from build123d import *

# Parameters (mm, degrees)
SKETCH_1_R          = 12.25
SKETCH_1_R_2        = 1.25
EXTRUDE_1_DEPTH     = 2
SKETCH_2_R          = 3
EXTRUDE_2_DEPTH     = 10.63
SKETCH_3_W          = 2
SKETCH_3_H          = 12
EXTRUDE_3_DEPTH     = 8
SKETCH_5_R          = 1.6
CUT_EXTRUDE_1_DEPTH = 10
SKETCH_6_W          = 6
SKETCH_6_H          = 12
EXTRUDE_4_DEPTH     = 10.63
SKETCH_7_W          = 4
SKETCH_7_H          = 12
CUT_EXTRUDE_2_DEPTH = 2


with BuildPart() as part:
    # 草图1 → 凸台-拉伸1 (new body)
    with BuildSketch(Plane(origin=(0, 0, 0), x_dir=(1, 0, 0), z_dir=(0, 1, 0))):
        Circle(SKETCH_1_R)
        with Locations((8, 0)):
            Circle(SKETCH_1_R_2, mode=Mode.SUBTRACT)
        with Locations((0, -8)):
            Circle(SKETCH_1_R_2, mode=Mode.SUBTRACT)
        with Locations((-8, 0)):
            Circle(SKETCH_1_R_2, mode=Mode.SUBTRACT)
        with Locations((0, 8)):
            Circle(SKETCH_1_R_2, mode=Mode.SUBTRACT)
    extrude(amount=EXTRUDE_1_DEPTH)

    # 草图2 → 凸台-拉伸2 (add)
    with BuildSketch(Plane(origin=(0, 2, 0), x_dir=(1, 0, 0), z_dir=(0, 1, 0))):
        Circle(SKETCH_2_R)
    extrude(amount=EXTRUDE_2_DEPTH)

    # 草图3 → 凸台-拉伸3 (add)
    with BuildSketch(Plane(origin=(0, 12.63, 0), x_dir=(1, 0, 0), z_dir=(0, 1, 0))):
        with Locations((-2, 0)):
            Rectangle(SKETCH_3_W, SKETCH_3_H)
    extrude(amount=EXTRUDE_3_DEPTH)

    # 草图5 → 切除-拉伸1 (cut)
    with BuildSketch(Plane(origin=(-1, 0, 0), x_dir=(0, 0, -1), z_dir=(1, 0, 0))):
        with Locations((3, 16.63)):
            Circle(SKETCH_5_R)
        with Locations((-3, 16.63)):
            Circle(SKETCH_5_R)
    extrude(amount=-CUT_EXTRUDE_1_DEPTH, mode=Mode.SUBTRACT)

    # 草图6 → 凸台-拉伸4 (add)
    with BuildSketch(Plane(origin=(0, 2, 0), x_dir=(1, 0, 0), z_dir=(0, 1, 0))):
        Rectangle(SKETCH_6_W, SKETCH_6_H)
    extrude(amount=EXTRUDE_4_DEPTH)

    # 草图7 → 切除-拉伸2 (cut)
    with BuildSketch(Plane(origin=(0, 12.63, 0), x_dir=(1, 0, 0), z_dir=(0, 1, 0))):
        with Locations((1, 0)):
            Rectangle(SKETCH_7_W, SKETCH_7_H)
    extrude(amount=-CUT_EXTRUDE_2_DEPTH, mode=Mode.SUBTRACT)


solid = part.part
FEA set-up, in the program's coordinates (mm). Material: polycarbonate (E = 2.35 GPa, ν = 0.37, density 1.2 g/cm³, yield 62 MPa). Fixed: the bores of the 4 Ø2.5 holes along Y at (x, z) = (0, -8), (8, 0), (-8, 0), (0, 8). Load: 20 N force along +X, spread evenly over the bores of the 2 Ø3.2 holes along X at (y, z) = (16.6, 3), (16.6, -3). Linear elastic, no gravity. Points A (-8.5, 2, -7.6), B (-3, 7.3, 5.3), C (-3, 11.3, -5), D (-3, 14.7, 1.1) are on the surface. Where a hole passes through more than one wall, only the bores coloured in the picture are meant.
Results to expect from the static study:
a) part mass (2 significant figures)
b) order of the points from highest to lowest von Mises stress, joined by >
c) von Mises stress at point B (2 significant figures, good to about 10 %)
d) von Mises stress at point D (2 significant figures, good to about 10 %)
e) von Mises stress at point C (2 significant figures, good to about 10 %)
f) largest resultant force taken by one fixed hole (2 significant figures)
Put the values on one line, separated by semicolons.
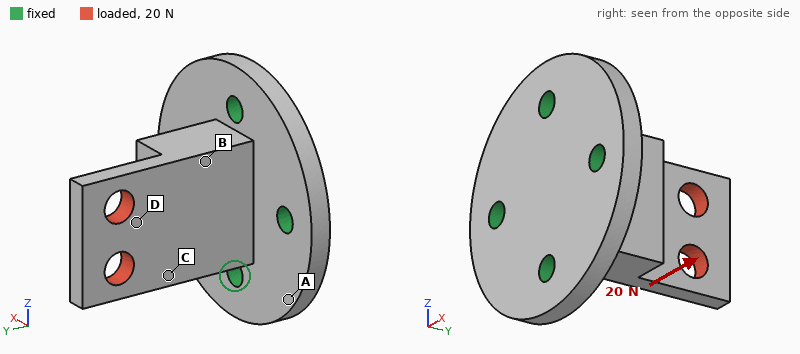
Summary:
2.1 g; C > D > B > A; 3.3 MPa; 6.1 MPa; 11 MPa; 20 N
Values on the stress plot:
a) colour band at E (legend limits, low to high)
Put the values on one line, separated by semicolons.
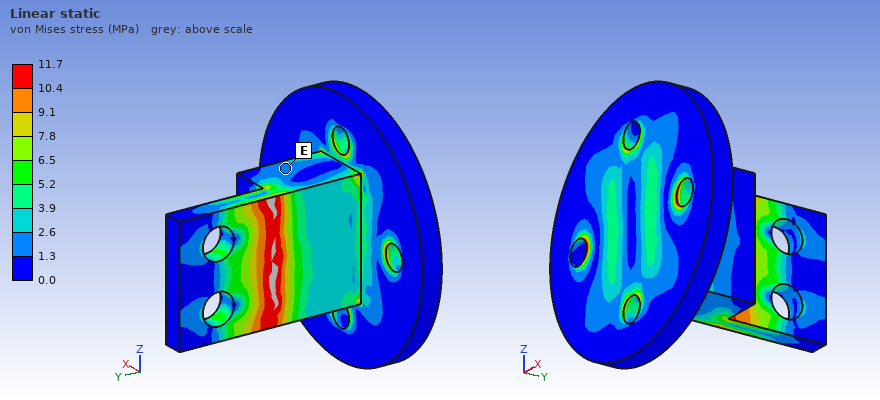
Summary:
1.3 to 2.6 MPa
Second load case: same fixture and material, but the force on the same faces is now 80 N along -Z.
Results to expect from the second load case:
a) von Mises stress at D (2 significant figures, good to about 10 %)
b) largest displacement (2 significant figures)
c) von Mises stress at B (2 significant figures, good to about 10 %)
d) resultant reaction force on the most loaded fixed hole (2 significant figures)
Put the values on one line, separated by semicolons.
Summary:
6.3 MPa; 0.24 mm; 8.9 MPa; 96 N
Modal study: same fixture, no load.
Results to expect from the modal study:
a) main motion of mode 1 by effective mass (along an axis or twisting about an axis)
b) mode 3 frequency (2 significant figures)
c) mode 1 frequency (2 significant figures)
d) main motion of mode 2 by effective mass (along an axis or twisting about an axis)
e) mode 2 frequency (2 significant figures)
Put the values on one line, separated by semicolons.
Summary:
along X; 6900 Hz; 3000 Hz; along Z; 6400 Hz
